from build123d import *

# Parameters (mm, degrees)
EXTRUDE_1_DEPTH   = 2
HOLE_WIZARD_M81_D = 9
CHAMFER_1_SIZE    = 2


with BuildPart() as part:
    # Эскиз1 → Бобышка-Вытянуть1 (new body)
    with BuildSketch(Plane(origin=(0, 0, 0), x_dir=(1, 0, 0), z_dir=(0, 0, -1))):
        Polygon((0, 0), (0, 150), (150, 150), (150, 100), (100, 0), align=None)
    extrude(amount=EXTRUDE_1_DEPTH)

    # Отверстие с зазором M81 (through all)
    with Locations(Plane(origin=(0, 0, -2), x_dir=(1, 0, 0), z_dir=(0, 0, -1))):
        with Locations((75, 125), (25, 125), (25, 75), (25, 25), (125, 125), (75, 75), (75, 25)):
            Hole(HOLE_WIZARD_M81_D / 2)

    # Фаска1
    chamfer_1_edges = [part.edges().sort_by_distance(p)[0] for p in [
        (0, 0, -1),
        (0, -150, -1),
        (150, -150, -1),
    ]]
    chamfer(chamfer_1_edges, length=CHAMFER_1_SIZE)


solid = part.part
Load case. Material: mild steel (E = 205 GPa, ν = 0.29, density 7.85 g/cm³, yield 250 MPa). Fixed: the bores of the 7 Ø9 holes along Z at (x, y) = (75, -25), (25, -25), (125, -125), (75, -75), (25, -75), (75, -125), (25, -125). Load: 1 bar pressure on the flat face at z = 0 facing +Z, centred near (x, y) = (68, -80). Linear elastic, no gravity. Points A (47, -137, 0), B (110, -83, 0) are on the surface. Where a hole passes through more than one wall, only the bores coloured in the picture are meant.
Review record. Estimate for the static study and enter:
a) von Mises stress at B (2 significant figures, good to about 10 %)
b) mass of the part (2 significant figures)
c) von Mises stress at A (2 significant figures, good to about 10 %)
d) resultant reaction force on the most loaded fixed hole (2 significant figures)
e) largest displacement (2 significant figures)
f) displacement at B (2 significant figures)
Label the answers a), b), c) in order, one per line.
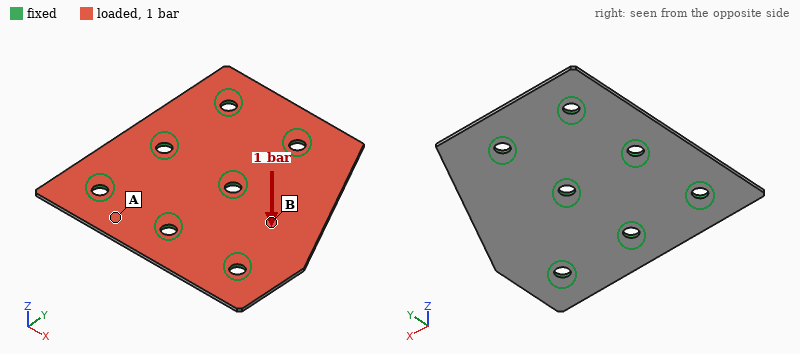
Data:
a) 43 MPa
b) 310 g
c) 16 MPa
d) 350 N
e) 0.33 mm
f) 0.13 mm
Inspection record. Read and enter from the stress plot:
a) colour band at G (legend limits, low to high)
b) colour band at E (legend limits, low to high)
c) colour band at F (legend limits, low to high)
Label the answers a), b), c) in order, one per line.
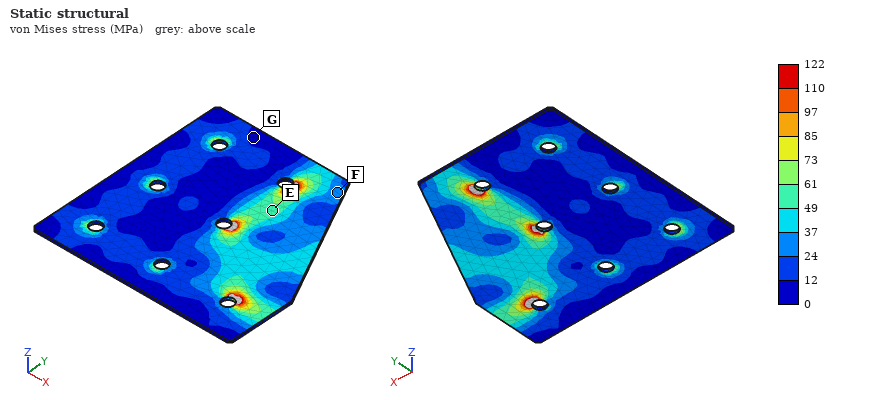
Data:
a) 0 to 12 MPa
b) 49 to 61 MPa
c) 24 to 37 MPa
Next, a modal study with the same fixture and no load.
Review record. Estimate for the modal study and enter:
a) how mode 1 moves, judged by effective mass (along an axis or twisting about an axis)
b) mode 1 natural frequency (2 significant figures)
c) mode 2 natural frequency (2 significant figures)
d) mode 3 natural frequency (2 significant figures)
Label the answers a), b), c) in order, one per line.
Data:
a) along Z
b) 950 Hz
c) 1800 Hz
d) 2500 Hz
